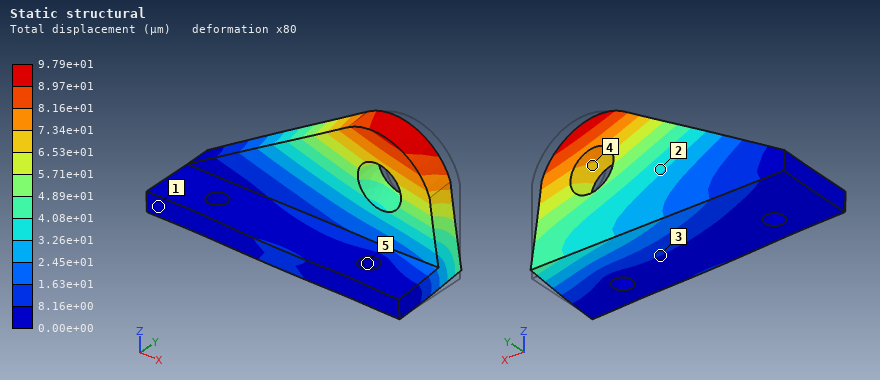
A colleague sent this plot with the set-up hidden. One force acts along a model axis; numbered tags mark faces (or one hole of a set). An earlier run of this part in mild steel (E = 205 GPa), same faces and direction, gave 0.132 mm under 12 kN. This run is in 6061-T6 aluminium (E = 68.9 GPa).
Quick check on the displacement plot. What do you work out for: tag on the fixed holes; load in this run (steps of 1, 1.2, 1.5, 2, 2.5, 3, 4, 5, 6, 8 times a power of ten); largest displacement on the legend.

5
3 kN
9.79e+01 µm
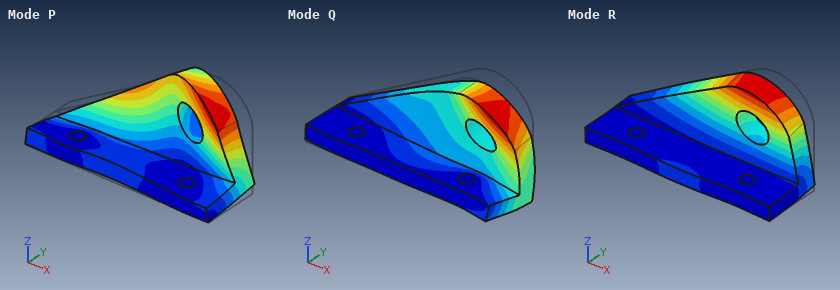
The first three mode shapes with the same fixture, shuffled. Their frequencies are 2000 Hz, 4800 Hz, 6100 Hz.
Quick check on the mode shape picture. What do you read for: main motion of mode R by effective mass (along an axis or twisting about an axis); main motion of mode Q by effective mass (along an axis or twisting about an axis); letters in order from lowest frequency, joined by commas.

along Y
along Z
R, P, Q
